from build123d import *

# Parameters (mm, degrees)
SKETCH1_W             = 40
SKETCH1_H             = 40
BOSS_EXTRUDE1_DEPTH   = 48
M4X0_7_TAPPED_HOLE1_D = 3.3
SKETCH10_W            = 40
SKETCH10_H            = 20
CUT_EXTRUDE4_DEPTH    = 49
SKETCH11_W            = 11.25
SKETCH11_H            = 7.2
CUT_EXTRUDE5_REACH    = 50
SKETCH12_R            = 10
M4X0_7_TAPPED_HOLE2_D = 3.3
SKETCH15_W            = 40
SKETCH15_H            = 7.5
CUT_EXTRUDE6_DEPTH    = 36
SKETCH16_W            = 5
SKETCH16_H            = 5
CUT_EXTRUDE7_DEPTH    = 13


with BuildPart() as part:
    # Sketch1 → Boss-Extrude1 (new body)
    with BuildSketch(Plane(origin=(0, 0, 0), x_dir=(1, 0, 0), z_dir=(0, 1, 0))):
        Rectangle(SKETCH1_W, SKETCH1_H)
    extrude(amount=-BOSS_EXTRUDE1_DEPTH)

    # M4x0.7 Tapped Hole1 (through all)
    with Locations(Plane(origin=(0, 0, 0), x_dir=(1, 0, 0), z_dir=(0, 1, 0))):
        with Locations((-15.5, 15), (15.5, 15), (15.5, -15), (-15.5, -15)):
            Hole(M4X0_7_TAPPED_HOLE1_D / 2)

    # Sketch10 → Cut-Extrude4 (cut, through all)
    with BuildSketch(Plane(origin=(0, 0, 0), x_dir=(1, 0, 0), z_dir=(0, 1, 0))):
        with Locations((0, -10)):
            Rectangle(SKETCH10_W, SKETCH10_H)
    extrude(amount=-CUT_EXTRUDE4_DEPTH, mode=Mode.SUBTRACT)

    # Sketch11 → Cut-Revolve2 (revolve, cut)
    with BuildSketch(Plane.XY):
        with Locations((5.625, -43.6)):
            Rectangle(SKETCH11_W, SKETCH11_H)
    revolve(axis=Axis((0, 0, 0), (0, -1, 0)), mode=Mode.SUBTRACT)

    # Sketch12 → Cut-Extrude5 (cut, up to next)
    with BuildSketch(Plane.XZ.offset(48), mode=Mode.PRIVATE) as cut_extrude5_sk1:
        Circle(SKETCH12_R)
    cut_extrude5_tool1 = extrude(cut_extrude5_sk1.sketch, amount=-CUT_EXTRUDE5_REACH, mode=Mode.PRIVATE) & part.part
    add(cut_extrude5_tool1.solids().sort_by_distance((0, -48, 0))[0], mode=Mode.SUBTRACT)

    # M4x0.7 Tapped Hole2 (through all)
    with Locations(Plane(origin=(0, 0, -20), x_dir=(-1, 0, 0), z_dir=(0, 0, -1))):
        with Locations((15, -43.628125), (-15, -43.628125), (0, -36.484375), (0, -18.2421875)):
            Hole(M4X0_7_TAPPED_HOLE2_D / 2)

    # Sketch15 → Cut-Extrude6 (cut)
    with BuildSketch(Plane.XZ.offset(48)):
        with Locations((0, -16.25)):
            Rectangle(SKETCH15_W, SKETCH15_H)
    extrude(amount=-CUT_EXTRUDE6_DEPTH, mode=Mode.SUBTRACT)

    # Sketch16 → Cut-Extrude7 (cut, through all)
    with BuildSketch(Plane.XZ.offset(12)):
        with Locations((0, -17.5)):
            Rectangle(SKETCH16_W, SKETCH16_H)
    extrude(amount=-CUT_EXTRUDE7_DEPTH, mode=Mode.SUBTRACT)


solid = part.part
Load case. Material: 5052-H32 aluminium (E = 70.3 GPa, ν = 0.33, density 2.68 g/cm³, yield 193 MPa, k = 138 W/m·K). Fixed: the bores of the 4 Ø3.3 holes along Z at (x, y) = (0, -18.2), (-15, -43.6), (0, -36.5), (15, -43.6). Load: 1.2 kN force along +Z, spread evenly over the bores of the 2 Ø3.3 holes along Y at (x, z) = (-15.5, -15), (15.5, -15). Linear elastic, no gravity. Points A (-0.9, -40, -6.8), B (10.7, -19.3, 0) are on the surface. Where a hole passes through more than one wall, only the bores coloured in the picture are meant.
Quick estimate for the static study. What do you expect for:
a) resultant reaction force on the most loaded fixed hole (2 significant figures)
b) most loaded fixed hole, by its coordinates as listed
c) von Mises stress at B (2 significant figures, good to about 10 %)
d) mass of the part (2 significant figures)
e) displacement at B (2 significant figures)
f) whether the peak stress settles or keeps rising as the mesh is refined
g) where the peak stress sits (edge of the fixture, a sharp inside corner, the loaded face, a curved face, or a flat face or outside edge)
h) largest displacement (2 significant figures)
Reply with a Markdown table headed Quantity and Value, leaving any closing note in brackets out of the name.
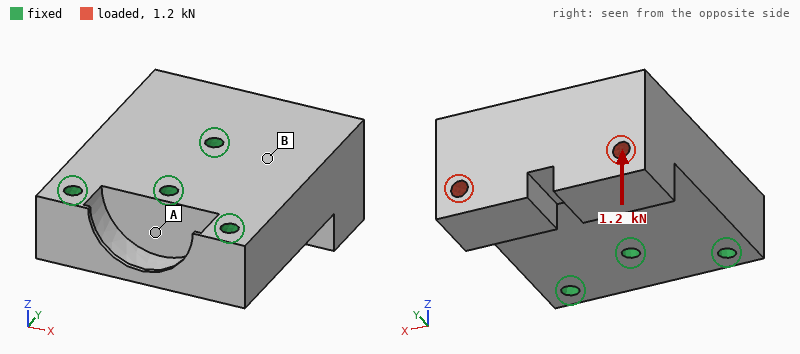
| Quantity | Value |
|---|---|
| resultant reaction force on the most loaded fixed hole | 1.4 kN |
| most loaded fixed hole, by its coordinates as listed | (0, -18.2) |
| von Mises stress at B | 7.6 MPa |
| mass of the part | 67 g |
| displacement at B | 2.3 µm |
| whether the peak stress settles or keeps rising as the mesh is refined | keeps rising |
| where the peak stress sits | edge of the fixture |
| largest displacement | 12 µm |
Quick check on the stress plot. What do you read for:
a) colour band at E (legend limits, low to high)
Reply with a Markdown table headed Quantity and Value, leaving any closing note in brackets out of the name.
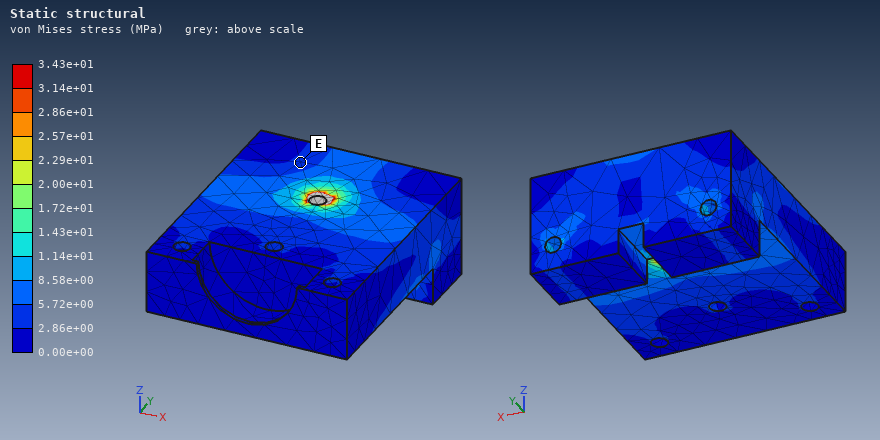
| Quantity | Value |
|---|---|
| colour band at E | 2.86e+00 to 5.72e+00 MPa |
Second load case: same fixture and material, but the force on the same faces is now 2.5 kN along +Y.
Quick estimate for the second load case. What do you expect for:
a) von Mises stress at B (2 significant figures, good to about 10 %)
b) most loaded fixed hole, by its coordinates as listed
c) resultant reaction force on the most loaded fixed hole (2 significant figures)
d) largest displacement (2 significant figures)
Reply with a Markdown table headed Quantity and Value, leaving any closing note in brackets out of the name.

| Quantity | Value |
|---|---|
| von Mises stress at B | 10 MPa |
| most loaded fixed hole, by its coordinates as listed | (0, -18.2) |
| resultant reaction force on the most loaded fixed hole | 1.4 kN |
| largest displacement | 19 µm |
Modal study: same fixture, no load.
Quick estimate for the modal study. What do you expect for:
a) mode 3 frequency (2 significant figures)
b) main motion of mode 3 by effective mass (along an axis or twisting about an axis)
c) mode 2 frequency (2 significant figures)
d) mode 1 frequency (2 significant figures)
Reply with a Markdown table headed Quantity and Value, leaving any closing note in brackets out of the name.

| Quantity | Value |
|---|---|
| mode 3 frequency | 19 kHz |
| main motion of mode 3 by effective mass | along X |
| mode 2 frequency | 13 kHz |
| mode 1 frequency | 13 kHz |
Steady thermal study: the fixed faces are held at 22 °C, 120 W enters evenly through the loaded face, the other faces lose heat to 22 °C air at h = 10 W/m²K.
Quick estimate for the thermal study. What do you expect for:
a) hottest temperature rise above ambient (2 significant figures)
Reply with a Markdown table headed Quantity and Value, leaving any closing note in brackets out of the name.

| Quantity | Value |
|---|---|
| hottest temperature rise above ambient | 53 K |
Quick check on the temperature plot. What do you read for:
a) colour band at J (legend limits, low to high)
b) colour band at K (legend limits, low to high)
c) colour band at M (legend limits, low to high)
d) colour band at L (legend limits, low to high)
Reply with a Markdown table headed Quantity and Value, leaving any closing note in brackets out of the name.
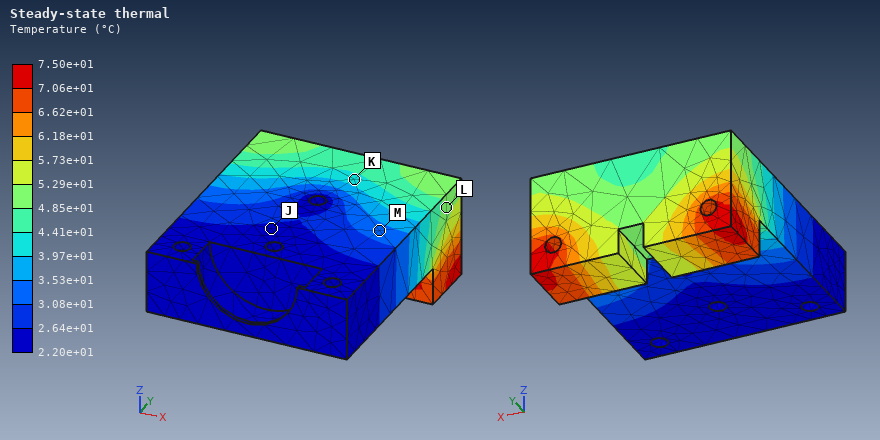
| Quantity | Value |
|---|---|
| colour band at J | 2.20e+01 to 2.64e+01 °C |
| colour band at K | 3.97e+01 to 4.41e+01 °C |
| colour band at M | 3.08e+01 to 3.53e+01 °C |
| colour band at L | 4.85e+01 to 5.29e+01 °C |
